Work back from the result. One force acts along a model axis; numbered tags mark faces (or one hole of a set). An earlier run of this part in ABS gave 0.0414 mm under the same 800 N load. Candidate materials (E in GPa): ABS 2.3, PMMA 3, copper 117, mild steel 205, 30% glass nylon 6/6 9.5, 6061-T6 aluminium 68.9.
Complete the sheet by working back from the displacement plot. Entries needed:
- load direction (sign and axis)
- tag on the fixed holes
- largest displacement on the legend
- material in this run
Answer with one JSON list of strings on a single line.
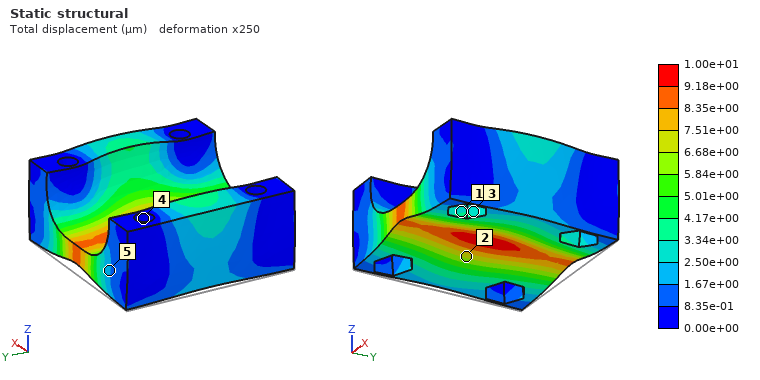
["+Z", "4", "1.00e+01 µm", "30% glass nylon 6/6"]
